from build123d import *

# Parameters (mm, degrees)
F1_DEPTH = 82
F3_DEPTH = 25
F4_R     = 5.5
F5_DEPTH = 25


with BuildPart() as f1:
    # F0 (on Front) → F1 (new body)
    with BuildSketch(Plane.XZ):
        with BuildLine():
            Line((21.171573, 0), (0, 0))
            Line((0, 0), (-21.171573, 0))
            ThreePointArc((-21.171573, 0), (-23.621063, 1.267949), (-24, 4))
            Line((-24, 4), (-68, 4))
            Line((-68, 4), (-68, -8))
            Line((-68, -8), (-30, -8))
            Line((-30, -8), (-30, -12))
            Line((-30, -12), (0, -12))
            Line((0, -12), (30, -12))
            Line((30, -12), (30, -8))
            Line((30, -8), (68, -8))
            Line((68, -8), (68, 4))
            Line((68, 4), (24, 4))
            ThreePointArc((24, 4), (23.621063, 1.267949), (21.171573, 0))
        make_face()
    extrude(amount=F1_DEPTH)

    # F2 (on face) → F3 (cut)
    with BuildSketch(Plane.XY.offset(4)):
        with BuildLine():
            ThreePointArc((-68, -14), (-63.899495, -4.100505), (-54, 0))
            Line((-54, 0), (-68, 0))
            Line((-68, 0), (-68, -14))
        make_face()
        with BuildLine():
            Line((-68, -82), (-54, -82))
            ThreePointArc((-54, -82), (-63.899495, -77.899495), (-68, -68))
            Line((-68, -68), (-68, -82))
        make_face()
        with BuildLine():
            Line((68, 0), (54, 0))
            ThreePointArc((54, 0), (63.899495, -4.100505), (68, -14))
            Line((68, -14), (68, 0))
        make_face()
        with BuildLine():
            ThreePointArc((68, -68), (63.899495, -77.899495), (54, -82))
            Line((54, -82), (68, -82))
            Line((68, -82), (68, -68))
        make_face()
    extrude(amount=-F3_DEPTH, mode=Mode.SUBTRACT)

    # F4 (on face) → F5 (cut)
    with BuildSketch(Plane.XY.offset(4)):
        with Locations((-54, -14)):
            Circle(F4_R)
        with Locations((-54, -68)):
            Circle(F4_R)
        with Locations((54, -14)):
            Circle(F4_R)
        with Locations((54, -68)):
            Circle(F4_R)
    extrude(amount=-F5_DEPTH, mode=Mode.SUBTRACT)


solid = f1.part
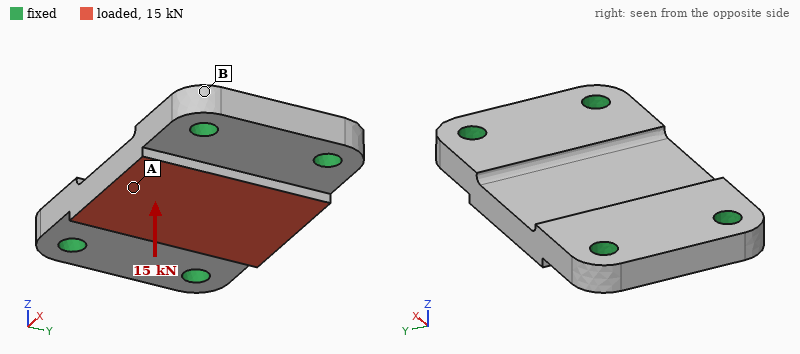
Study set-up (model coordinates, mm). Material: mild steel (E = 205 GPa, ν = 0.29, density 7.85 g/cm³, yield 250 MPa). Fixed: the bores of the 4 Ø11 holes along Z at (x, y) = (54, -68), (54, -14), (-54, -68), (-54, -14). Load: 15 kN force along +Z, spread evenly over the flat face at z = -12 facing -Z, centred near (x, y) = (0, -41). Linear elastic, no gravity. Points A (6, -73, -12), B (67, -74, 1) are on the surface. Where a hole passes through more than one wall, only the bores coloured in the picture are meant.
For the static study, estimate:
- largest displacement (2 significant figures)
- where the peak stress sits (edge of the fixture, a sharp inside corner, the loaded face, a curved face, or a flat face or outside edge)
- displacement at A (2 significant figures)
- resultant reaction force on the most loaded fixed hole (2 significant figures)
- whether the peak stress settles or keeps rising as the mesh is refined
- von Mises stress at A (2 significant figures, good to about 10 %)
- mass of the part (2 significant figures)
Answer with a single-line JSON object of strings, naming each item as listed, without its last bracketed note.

{"largest displacement": "29 µm", "where the peak stress sits": "edge of the fixture", "displacement at A": "28 µm", "resultant reaction force on the most loaded fixed hole": "6.0 kN", "whether the peak stress settles or keeps rising as the mesh is refined": "keeps rising", "von Mises stress at A": "52 MPa", "mass of the part": "1.0 kg"}
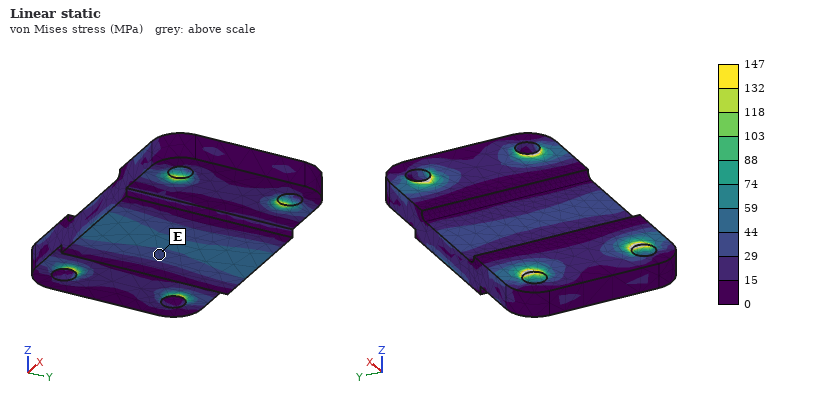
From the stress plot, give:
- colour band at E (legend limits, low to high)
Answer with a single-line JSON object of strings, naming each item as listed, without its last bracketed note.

{"colour band at E": "29 to 44 MPa"}
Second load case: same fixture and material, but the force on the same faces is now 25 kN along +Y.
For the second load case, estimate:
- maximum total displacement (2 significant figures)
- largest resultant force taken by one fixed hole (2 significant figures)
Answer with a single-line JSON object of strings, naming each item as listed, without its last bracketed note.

{"maximum total displacement": "24 µm", "largest resultant force taken by one fixed hole": "8.8 kN"}
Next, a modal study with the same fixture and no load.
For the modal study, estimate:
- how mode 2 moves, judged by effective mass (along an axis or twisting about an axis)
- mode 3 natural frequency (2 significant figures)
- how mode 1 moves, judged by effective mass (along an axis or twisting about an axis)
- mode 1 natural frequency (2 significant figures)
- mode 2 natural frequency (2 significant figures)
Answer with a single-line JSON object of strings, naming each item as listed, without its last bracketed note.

{"how mode 2 moves, judged by effective mass": "twisting about X", "mode 3 natural frequency": "12 kHz", "how mode 1 moves, judged by effective mass": "along Z", "mode 1 natural frequency": "5500 Hz", "mode 2 natural frequency": "7100 Hz"}
